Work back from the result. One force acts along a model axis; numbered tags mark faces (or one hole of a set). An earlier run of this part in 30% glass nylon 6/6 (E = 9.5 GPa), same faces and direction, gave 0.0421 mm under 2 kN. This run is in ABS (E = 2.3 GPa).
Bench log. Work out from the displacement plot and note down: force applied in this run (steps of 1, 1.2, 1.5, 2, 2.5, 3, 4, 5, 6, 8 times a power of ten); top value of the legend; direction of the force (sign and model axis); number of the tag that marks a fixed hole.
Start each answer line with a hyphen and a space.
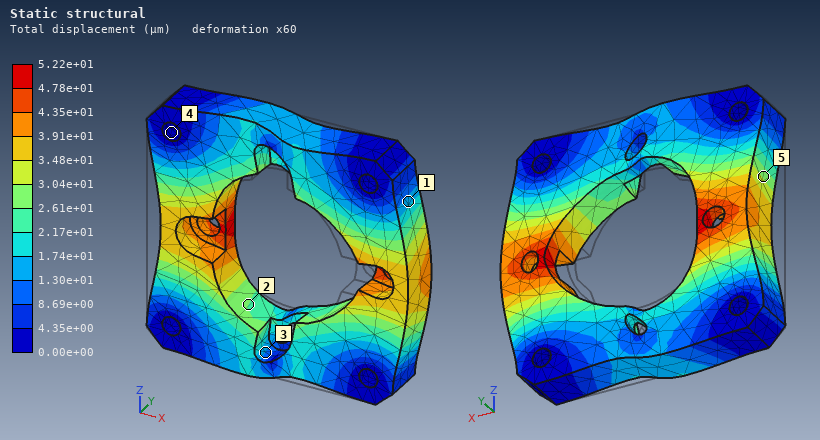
- 600 N
- 5.22e+01 µm
- +X
- 4
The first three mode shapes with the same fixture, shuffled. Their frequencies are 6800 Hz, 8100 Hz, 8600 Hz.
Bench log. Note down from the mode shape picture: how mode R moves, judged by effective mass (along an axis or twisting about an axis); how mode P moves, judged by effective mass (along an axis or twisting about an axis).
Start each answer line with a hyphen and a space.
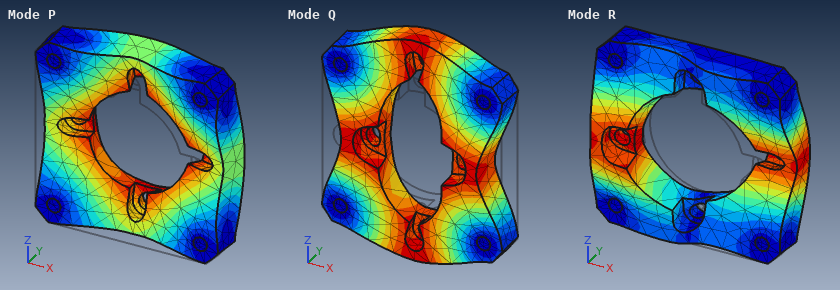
- twisting about Z
- along Y
